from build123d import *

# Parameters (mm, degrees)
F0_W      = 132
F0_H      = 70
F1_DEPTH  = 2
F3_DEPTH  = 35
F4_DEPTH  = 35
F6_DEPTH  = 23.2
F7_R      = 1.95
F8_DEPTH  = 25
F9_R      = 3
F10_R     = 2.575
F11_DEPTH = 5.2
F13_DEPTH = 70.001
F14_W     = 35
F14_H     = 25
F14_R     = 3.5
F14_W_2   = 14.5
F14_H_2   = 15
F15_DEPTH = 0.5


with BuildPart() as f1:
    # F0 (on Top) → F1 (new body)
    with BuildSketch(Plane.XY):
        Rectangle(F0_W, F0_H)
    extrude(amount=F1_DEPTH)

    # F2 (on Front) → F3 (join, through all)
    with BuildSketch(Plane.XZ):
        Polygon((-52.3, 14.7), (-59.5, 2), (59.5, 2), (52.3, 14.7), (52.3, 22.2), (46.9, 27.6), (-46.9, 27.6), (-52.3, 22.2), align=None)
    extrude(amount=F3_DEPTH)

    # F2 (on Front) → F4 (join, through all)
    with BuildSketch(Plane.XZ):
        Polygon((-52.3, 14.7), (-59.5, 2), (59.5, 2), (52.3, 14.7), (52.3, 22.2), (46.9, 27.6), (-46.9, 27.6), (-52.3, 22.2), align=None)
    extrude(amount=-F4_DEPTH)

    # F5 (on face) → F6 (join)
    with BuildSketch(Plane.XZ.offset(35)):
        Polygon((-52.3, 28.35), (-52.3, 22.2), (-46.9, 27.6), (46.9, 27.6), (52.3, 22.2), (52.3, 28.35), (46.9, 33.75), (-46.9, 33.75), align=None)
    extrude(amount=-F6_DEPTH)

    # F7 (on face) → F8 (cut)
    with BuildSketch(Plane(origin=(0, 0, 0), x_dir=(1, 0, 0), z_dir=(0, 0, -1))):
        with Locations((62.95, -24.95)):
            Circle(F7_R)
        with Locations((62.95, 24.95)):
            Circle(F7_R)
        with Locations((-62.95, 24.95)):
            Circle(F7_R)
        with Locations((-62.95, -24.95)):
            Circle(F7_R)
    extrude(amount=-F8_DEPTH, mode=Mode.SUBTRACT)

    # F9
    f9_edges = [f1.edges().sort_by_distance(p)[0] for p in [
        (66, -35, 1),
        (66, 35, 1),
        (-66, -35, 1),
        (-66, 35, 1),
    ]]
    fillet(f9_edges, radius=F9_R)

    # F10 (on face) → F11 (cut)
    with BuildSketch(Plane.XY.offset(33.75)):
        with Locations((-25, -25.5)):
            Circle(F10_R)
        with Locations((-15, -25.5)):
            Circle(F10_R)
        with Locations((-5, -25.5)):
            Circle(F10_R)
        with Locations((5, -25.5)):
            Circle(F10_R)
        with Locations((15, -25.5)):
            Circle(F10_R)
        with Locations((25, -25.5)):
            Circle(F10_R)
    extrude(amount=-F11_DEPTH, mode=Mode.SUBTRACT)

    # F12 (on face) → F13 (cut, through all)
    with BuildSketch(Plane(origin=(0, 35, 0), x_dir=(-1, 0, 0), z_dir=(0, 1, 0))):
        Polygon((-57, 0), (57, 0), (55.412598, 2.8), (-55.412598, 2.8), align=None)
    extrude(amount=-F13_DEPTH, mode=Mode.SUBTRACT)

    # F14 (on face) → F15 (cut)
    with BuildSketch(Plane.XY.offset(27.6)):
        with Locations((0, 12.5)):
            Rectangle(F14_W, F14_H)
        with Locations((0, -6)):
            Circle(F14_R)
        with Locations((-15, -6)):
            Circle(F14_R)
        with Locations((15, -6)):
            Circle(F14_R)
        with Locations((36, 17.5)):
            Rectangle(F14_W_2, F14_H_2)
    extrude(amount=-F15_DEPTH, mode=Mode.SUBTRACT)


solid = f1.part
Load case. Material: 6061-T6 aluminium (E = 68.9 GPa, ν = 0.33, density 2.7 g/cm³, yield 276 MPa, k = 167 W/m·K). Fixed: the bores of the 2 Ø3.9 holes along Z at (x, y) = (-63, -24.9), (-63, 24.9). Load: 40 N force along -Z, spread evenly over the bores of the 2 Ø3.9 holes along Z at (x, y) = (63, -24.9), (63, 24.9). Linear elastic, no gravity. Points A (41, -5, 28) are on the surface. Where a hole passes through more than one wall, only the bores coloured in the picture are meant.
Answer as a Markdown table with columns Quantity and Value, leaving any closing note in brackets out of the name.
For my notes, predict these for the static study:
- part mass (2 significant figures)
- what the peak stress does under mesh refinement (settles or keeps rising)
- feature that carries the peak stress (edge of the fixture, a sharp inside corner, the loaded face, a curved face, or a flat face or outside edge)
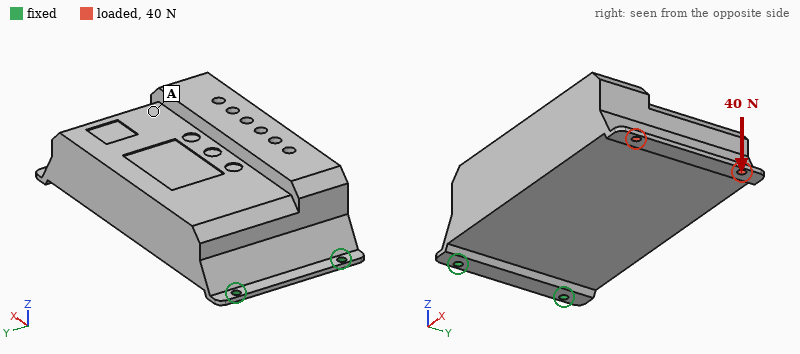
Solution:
| Quantity | Value |
|---|---|
| part mass | 540 g |
| what the peak stress does under mesh refinement | keeps rising |
| feature that carries the peak stress | edge of the fixture |
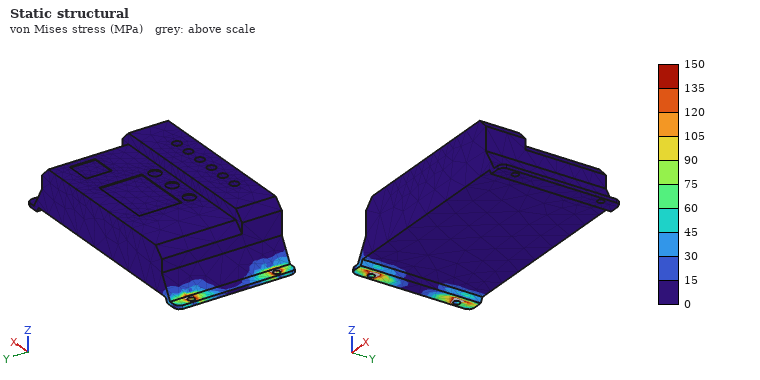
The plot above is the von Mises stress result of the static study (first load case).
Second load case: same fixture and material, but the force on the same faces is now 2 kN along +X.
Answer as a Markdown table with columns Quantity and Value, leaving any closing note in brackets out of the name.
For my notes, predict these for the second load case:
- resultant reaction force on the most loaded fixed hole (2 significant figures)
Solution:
| Quantity | Value |
|---|---|
| resultant reaction force on the most loaded fixed hole | 1.0 kN |
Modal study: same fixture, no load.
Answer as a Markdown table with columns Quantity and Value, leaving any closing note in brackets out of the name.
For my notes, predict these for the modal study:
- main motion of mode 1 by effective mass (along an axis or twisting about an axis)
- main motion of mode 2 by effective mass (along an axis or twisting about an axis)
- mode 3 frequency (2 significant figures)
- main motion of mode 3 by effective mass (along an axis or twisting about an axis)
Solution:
| Quantity | Value |
|---|---|
| main motion of mode 1 by effective mass | along Z |
| main motion of mode 2 by effective mass | along Y |
| mode 3 frequency | 1800 Hz |
| main motion of mode 3 by effective mass | along Y |
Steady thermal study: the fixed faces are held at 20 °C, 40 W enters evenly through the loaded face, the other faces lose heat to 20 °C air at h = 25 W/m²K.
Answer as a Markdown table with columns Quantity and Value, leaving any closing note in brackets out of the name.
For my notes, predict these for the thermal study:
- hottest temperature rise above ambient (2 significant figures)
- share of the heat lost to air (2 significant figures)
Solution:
| Quantity | Value |
|---|---|
| hottest temperature rise above ambient | 69 K |
| share of the heat lost to air | 41 % |
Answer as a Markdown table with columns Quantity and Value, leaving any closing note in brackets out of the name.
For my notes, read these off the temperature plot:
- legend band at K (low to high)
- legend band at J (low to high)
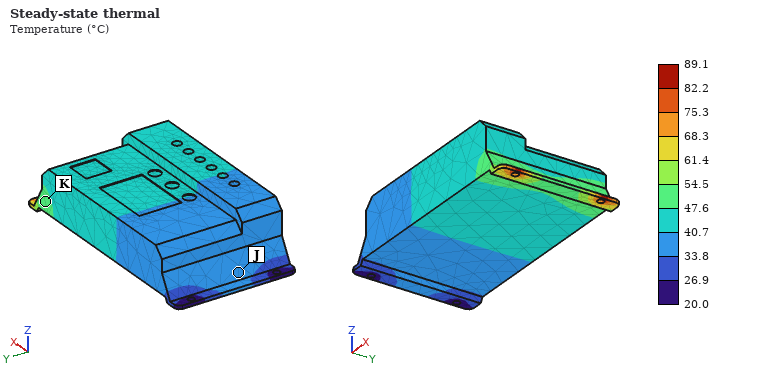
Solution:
| Quantity | Value |
|---|---|
| legend band at K | 47.6 to 54.5 °C |
| legend band at J | 33.8 to 40.7 °C |
